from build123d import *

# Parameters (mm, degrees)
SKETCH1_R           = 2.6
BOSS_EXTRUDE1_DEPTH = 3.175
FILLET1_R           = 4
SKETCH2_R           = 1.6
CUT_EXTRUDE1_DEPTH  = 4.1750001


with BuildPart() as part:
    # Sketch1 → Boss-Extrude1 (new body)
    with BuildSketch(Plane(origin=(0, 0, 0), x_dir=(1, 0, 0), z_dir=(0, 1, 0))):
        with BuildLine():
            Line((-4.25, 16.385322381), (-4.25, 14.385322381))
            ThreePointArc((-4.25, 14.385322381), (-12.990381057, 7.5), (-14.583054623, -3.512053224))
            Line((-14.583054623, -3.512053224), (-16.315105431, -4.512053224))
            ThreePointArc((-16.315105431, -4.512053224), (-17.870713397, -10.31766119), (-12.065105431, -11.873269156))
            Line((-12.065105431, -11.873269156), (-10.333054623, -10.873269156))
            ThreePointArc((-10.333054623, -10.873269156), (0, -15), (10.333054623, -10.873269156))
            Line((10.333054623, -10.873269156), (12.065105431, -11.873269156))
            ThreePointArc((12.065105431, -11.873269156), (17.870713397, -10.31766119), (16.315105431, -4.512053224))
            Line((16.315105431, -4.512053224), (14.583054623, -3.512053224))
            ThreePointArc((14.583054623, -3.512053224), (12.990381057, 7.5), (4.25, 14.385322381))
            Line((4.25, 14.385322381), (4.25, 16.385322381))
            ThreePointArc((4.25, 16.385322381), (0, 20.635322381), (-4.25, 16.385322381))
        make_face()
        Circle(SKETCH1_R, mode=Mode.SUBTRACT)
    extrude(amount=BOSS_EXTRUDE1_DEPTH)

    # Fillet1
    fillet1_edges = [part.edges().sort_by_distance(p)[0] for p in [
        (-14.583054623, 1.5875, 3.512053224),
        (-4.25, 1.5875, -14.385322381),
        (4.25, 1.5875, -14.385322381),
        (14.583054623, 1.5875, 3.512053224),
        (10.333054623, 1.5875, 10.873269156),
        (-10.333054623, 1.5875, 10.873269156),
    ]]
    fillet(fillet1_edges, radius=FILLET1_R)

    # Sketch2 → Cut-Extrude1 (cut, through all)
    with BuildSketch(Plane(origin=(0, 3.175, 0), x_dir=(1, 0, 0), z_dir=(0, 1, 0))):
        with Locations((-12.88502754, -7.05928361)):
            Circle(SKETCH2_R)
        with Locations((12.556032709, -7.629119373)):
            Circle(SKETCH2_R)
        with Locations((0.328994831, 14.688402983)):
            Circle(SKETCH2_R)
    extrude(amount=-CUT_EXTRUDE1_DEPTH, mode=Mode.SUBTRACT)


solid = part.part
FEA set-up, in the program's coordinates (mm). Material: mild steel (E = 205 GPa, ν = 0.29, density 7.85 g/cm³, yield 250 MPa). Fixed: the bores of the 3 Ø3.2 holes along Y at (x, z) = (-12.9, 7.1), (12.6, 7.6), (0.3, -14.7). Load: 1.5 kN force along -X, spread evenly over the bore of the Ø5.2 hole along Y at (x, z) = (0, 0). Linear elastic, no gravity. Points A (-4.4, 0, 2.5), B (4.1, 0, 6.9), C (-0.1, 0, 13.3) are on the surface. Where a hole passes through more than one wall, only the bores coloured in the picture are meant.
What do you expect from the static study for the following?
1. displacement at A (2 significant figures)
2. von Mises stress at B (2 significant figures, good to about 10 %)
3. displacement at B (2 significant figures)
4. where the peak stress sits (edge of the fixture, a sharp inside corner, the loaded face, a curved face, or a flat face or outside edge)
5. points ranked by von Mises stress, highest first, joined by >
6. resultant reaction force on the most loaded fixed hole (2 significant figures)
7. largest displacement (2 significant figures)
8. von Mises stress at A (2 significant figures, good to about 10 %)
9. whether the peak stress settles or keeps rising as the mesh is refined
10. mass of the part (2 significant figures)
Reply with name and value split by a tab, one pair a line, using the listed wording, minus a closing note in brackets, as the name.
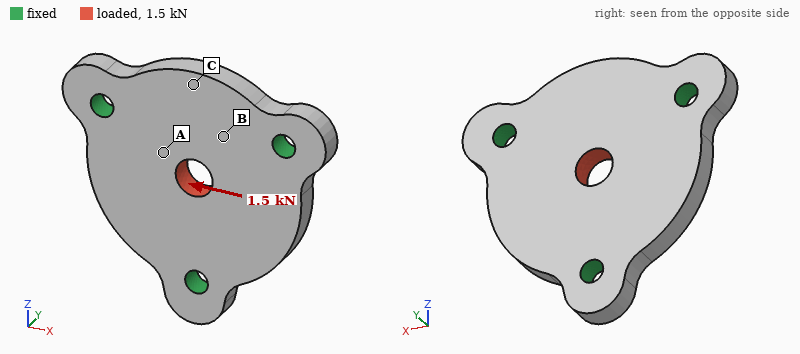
displacement at A	1.1 µm
von Mises stress at B	15 MPa
displacement at B	0.60 µm
where the peak stress sits	edge of the fixture
points ranked by von Mises stress, highest first, joined by >	A > B > C
resultant reaction force on the most loaded fixed hole	570 N
largest displacement	2.0 µm
von Mises stress at A	27 MPa
whether the peak stress settles or keeps rising as the mesh is refined	keeps rising
mass of the part	20 g
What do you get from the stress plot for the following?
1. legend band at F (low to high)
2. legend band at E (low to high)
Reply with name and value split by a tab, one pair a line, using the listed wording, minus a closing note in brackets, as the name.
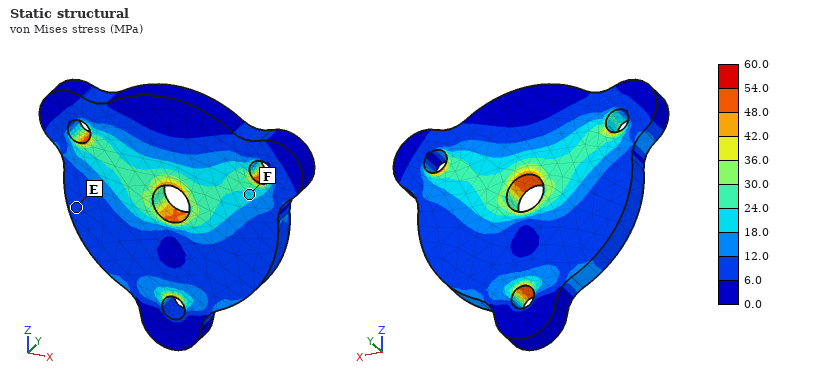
legend band at F	18.0 to 24.0 MPa
legend band at E	6.0 to 12.0 MPa
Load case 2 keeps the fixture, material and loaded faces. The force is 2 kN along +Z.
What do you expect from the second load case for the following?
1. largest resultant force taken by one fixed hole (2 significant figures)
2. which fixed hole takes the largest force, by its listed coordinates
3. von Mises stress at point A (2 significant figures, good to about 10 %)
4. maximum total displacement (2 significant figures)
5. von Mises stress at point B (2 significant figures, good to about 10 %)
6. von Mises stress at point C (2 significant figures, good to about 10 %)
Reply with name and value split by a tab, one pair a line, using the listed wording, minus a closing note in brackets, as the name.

largest resultant force taken by one fixed hole	830 N
which fixed hole takes the largest force, by its listed coordinates	(0.3, -14.7)
von Mises stress at point A	21 MPa
maximum total displacement	2.7 µm
von Mises stress at point B	19 MPa
von Mises stress at point C	16 MPa
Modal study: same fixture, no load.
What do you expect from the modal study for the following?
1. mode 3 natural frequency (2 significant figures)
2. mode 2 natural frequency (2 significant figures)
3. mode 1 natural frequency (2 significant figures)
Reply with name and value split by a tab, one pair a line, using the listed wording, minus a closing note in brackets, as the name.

mode 3 natural frequency	23 kHz
mode 2 natural frequency	23 kHz
mode 1 natural frequency	22 kHz
